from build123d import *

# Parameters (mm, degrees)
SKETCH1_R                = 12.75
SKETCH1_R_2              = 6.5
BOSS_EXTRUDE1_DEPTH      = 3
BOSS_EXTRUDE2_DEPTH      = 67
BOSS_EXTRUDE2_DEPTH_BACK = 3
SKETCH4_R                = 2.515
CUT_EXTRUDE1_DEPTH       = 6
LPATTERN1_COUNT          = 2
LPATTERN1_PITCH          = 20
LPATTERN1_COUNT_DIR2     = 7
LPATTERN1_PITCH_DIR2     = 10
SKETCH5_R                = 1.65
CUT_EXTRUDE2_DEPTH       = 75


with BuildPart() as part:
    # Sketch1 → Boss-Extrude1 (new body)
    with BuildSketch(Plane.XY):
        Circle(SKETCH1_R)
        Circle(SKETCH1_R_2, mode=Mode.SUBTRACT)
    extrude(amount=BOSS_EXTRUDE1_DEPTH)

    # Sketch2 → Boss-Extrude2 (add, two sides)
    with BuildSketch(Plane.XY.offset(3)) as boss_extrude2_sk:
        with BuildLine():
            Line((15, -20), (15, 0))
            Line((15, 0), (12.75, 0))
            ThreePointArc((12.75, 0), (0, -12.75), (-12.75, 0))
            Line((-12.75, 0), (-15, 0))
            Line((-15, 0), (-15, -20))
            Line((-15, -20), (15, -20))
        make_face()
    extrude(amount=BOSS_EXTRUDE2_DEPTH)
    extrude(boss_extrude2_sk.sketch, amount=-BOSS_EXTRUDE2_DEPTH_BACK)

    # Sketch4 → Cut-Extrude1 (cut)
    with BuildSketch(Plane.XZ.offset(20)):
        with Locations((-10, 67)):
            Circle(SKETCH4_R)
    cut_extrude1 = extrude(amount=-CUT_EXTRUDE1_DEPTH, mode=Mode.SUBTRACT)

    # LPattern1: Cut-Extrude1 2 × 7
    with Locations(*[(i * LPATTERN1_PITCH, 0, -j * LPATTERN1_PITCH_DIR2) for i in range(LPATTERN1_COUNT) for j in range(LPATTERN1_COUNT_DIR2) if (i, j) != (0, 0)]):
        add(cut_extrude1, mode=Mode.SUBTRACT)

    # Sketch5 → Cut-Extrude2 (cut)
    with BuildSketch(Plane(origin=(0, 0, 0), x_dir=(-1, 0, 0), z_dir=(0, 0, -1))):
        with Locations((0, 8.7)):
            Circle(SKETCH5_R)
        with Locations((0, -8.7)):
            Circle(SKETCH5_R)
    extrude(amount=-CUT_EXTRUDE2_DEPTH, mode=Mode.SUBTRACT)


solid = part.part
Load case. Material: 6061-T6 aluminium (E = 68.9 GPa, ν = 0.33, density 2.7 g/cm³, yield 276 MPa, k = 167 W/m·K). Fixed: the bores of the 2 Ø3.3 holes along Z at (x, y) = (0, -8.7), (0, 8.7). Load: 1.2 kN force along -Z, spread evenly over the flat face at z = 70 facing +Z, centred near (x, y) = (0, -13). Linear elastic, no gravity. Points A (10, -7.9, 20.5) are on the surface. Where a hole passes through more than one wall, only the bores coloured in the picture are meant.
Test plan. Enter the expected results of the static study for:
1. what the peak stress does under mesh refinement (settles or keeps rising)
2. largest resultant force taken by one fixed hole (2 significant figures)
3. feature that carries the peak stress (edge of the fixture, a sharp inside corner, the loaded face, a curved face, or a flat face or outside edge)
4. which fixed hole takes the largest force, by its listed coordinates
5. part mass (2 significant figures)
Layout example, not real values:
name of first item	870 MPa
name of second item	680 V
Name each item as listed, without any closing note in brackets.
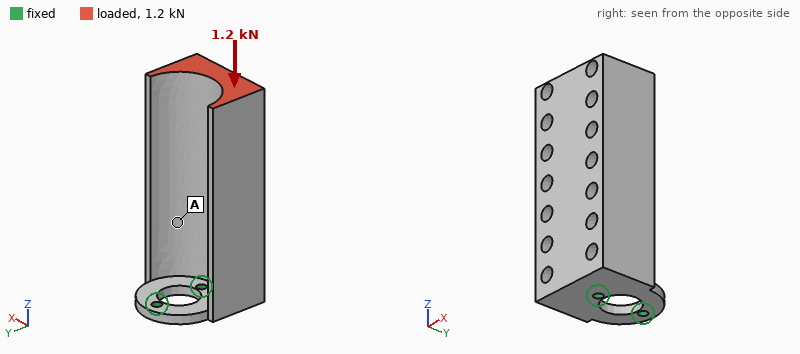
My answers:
what the peak stress does under mesh refinement	keeps rising
largest resultant force taken by one fixed hole	1.3 kN
feature that carries the peak stress	edge of the fixture
which fixed hole takes the largest force, by its listed coordinates	(0, -8.7)
part mass	64 g
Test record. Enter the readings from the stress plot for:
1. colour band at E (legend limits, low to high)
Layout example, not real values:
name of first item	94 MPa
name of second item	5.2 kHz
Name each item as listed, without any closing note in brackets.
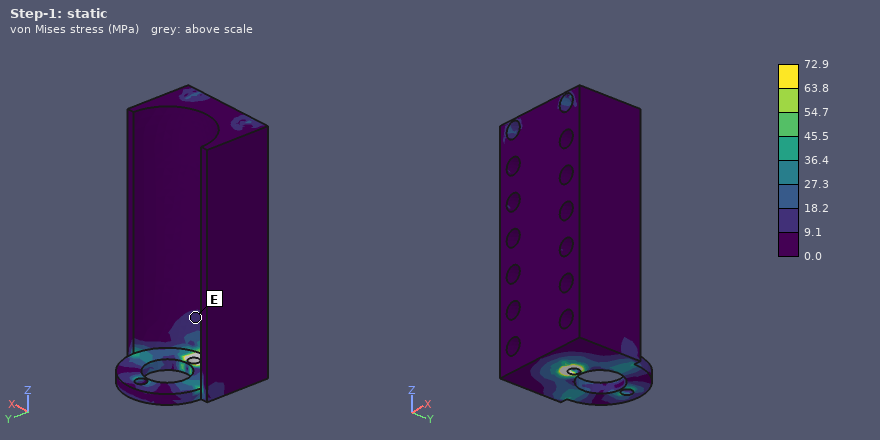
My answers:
colour band at E	9.1 to 18.2 MPa
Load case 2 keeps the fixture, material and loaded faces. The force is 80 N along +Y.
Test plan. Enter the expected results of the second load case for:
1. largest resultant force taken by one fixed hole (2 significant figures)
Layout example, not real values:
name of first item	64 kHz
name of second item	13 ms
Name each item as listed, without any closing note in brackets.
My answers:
largest resultant force taken by one fixed hole	190 N
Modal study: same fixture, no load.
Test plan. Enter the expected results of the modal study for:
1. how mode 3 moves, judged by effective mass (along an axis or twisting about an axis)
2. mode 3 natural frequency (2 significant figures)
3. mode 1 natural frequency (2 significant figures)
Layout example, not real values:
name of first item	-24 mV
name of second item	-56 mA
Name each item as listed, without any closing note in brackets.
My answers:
how mode 3 moves, judged by effective mass	twisting about Z
mode 3 natural frequency	3900 Hz
mode 1 natural frequency	620 Hz
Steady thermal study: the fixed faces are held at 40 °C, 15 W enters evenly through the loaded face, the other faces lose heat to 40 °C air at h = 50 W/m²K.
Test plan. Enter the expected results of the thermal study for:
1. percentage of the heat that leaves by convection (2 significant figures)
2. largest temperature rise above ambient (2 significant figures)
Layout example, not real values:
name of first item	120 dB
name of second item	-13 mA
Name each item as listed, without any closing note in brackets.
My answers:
percentage of the heat that leaves by convection	39 %
largest temperature rise above ambient	22 K
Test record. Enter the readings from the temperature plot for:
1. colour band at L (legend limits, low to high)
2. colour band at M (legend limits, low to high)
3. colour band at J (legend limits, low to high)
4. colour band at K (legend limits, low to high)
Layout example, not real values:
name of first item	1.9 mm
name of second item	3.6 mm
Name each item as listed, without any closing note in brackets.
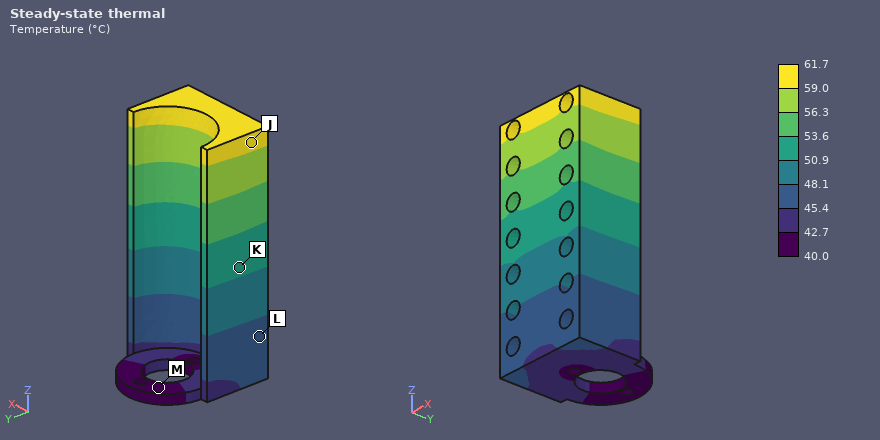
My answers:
colour band at L	45.4 to 48.1 °C
colour band at M	40.0 to 42.7 °C
colour band at J	59.0 to 61.7 °C
colour band at K	50.9 to 53.6 °C
